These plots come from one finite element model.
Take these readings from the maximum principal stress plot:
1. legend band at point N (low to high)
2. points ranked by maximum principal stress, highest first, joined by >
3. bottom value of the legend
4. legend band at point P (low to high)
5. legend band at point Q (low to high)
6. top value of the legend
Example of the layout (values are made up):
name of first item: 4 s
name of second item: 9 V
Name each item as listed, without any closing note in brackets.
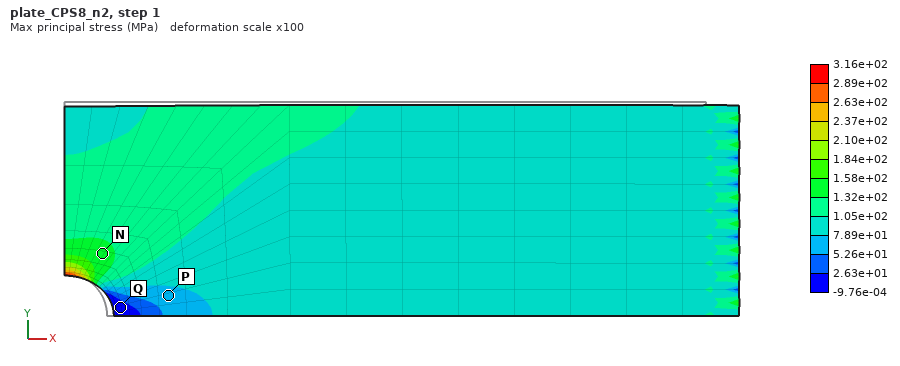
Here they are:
legend band at point N: 1.32e+02 to 1.58e+02 MPa
points ranked by maximum principal stress, highest first, joined by >: N > P > Q
bottom value of the legend: -9.76e-04 MPa
legend band at point P: 5.26e+01 to 7.89e+01 MPa
legend band at point Q: -9.76e-04 to 2.63e+01 MPa
top value of the legend: 3.16e+02 MPa
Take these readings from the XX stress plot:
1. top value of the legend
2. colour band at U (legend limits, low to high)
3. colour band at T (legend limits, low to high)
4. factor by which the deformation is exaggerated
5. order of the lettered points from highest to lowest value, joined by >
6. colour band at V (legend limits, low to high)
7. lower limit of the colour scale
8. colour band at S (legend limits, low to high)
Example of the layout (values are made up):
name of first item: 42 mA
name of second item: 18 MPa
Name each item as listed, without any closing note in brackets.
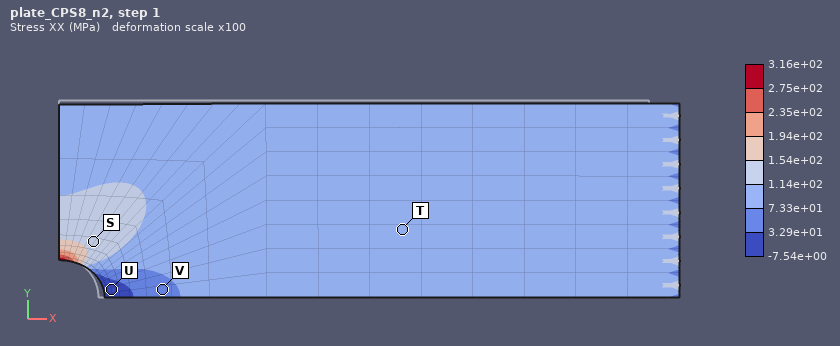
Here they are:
top value of the legend: 3.16e+02 MPa
colour band at U: -7.54e+00 to 3.29e+01 MPa
colour band at T: 7.33e+01 to 1.14e+02 MPa
factor by which the deformation is exaggerated: 100
order of the lettered points from highest to lowest value, joined by >: S > T > V > U
colour band at V: 3.29e+01 to 7.33e+01 MPa
lower limit of the colour scale: -7.54e+00 MPa
colour band at S: 1.14e+02 to 1.54e+02 MPa
